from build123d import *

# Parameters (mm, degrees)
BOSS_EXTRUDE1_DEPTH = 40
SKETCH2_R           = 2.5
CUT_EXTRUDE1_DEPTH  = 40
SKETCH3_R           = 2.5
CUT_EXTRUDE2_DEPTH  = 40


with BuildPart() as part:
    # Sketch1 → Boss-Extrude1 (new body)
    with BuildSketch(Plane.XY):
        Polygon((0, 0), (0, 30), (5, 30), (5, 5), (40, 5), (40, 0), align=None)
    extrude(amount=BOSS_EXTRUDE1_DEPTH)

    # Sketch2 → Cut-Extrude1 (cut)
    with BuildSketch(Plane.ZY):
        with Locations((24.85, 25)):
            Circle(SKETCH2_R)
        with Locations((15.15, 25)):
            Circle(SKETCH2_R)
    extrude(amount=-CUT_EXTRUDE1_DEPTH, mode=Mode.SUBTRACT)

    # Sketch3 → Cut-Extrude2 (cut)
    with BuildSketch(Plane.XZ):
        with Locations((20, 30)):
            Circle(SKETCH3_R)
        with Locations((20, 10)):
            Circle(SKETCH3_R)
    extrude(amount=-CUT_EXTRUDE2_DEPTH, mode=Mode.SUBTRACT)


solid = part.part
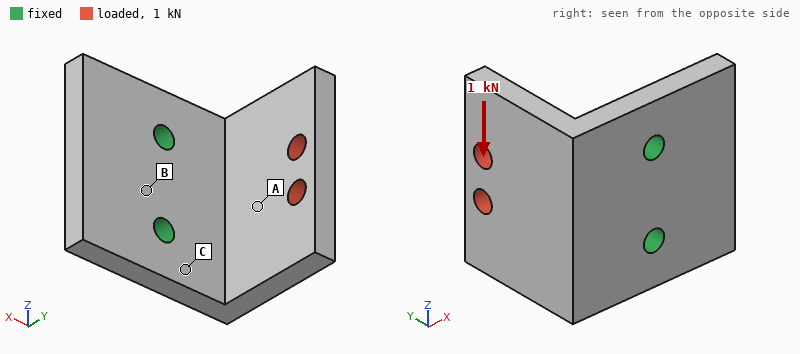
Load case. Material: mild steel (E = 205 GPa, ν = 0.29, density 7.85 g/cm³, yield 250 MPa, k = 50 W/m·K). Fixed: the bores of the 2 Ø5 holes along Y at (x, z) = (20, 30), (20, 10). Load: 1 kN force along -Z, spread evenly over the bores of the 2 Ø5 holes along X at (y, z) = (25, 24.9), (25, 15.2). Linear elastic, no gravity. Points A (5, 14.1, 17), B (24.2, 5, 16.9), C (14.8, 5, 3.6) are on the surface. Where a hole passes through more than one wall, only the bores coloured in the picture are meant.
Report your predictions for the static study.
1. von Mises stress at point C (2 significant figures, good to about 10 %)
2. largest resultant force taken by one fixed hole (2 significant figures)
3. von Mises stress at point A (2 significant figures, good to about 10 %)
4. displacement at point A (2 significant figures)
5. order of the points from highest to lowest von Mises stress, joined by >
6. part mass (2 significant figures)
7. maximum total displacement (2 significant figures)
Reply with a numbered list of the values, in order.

1. 55 MPa
2. 1.2 kN
3. 29 MPa
4. 17 µm
5. C > A > B
6. 99 g
7. 46 µm
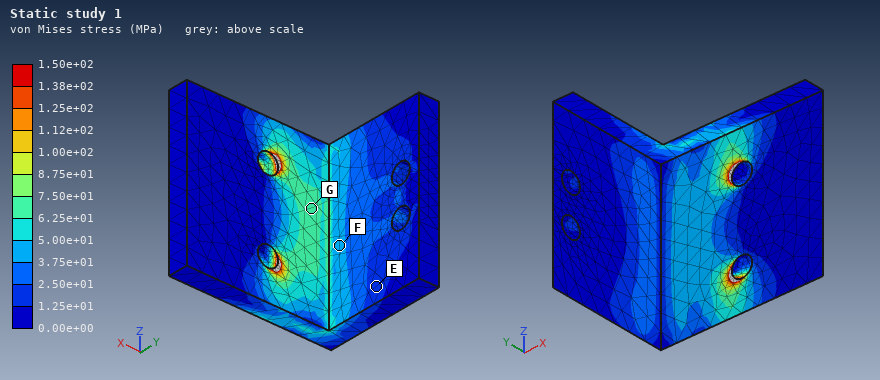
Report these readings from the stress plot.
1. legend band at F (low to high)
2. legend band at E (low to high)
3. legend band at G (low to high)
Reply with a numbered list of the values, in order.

1. 3.75e+01 to 5.00e+01 MPa
2. 1.25e+01 to 2.50e+01 MPa
3. 6.25e+01 to 7.50e+01 MPa
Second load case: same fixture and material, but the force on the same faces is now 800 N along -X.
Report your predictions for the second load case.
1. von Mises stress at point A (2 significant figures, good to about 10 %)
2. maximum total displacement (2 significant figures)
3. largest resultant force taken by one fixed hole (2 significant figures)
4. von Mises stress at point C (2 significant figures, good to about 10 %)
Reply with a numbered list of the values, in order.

1. 54 MPa
2. 0.14 mm
3. 420 N
4. 91 MPa
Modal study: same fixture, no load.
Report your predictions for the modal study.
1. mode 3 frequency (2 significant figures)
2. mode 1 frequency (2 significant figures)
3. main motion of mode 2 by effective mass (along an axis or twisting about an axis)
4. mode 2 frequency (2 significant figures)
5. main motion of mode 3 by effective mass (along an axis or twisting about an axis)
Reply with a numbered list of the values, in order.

1. 8200 Hz
2. 2800 Hz
3. along Z
4. 5000 Hz
5. along Y
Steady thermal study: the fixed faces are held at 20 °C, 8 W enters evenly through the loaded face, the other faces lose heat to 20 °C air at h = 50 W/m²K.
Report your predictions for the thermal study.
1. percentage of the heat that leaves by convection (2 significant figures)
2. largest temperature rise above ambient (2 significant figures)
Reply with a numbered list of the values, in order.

1. 33 %
2. 29 K
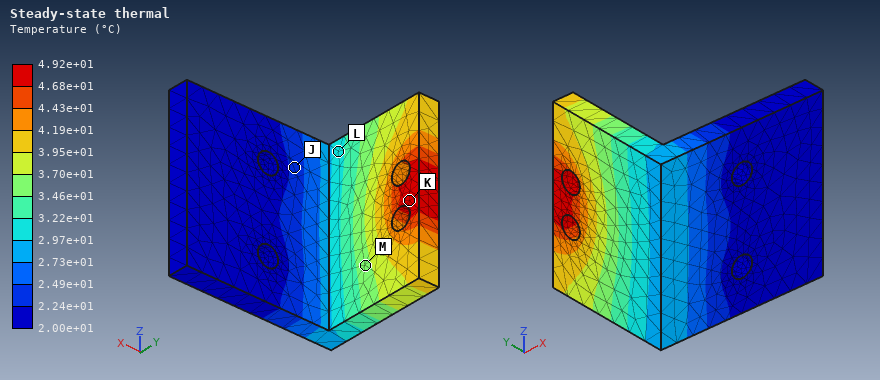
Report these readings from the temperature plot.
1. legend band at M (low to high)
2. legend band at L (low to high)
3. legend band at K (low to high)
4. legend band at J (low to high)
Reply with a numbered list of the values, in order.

1. 3.46e+01 to 3.70e+01 °C
2. 2.97e+01 to 3.22e+01 °C
3. 4.68e+01 to 4.92e+01 °C
4. 2.24e+01 to 2.49e+01 °C
